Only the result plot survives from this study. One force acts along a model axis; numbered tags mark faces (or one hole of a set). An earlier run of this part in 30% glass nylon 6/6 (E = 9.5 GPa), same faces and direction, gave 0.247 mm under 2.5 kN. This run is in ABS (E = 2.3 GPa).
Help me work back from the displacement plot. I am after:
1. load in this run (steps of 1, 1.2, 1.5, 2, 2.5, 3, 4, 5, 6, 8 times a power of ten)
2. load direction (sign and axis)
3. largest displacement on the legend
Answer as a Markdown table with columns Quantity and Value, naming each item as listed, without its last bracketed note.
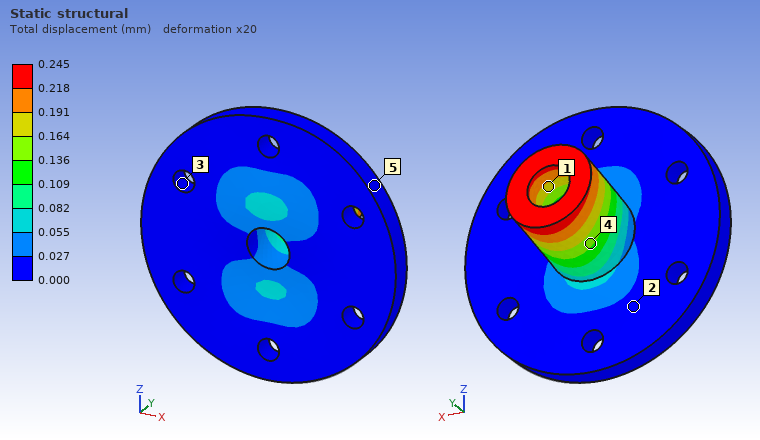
| Quantity | Value |
|---|---|
| load in this run | 600 N |
| load direction | +Z |
| largest displacement on the legend | 0.245 mm |
